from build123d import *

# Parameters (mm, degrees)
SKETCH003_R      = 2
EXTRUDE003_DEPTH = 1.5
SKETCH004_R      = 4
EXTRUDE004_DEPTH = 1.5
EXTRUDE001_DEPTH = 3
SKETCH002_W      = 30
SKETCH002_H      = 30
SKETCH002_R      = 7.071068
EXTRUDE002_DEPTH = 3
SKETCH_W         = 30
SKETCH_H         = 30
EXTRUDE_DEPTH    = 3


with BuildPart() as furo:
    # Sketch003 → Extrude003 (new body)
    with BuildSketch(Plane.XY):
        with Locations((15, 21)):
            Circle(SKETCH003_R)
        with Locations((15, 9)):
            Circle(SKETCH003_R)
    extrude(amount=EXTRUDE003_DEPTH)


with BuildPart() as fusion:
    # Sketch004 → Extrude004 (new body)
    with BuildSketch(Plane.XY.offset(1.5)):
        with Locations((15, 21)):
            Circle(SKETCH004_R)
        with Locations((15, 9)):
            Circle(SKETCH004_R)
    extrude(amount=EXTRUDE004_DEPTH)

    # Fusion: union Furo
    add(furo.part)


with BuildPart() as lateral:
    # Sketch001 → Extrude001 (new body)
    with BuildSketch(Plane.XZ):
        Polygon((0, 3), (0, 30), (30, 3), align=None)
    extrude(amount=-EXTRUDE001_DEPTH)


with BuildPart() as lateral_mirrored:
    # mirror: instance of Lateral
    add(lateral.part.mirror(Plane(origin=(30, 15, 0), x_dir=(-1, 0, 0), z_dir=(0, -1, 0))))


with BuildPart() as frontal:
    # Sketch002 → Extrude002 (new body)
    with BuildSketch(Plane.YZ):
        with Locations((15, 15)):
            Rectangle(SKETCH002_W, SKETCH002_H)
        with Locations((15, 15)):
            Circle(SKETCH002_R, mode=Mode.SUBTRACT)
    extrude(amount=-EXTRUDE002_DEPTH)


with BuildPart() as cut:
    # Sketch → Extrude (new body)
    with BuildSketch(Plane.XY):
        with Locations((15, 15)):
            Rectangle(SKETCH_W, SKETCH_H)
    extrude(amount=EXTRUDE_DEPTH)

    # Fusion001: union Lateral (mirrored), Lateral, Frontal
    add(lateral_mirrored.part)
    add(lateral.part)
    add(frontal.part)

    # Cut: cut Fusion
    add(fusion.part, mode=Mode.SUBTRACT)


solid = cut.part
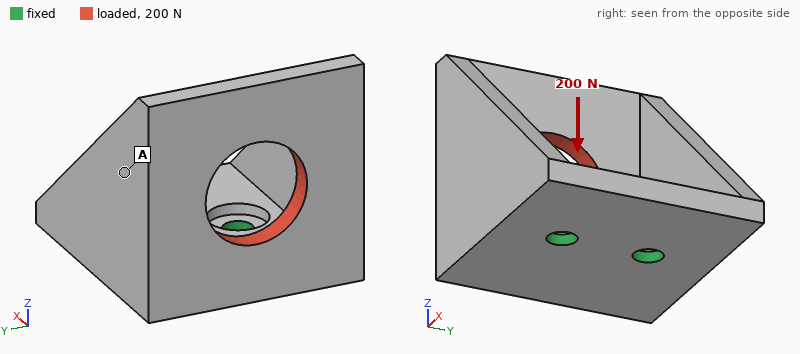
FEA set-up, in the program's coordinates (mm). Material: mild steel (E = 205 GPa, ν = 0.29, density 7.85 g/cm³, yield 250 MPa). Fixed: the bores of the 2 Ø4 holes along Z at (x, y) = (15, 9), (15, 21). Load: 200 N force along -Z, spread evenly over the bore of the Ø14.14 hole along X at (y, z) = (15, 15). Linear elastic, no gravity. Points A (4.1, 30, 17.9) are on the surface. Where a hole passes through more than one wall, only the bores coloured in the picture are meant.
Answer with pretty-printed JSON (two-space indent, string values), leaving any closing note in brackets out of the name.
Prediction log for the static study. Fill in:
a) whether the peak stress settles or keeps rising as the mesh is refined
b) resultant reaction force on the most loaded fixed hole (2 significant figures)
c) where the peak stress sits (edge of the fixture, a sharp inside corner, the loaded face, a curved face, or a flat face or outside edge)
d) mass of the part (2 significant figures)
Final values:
{
  "whether the peak stress settles or keeps rising as the mesh is refined": "keeps rising",
  "resultant reaction force on the most loaded fixed hole": "110 N",
  "where the peak stress sits": "edge of the fixture",
  "mass of the part": "56 g"
}
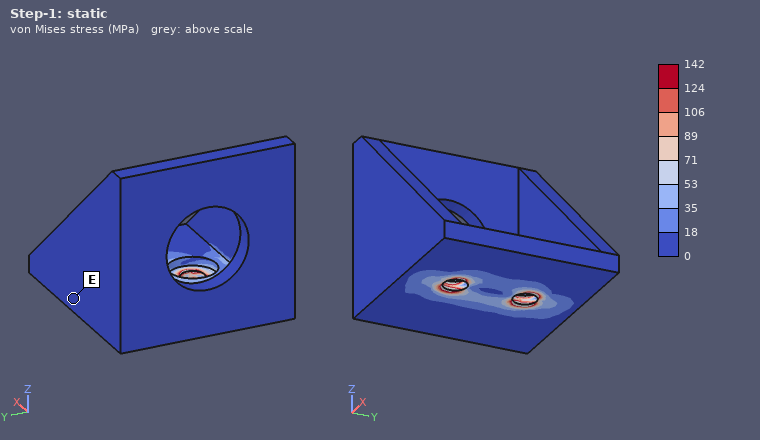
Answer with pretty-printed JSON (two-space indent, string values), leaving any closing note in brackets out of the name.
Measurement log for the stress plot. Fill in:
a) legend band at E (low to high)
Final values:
{
  "legend band at E": "0 to 18 MPa"
}
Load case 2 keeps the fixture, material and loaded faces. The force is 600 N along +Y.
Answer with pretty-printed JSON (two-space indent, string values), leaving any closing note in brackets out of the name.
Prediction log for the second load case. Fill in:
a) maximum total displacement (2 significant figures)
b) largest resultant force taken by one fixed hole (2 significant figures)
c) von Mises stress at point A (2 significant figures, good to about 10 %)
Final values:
{
  "maximum total displacement": "69 µm",
  "largest resultant force taken by one fixed hole": "930 N",
  "von Mises stress at point A": "22 MPa"
}
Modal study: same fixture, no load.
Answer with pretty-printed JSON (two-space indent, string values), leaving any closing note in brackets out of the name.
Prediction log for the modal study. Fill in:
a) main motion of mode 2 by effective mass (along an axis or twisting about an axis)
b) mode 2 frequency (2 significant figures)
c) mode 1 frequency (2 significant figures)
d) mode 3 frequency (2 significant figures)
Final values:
{
  "main motion of mode 2 by effective mass": "along Y",
  "mode 2 frequency": "2900 Hz",
  "mode 1 frequency": "2000 Hz",
  "mode 3 frequency": "7800 Hz"
}
